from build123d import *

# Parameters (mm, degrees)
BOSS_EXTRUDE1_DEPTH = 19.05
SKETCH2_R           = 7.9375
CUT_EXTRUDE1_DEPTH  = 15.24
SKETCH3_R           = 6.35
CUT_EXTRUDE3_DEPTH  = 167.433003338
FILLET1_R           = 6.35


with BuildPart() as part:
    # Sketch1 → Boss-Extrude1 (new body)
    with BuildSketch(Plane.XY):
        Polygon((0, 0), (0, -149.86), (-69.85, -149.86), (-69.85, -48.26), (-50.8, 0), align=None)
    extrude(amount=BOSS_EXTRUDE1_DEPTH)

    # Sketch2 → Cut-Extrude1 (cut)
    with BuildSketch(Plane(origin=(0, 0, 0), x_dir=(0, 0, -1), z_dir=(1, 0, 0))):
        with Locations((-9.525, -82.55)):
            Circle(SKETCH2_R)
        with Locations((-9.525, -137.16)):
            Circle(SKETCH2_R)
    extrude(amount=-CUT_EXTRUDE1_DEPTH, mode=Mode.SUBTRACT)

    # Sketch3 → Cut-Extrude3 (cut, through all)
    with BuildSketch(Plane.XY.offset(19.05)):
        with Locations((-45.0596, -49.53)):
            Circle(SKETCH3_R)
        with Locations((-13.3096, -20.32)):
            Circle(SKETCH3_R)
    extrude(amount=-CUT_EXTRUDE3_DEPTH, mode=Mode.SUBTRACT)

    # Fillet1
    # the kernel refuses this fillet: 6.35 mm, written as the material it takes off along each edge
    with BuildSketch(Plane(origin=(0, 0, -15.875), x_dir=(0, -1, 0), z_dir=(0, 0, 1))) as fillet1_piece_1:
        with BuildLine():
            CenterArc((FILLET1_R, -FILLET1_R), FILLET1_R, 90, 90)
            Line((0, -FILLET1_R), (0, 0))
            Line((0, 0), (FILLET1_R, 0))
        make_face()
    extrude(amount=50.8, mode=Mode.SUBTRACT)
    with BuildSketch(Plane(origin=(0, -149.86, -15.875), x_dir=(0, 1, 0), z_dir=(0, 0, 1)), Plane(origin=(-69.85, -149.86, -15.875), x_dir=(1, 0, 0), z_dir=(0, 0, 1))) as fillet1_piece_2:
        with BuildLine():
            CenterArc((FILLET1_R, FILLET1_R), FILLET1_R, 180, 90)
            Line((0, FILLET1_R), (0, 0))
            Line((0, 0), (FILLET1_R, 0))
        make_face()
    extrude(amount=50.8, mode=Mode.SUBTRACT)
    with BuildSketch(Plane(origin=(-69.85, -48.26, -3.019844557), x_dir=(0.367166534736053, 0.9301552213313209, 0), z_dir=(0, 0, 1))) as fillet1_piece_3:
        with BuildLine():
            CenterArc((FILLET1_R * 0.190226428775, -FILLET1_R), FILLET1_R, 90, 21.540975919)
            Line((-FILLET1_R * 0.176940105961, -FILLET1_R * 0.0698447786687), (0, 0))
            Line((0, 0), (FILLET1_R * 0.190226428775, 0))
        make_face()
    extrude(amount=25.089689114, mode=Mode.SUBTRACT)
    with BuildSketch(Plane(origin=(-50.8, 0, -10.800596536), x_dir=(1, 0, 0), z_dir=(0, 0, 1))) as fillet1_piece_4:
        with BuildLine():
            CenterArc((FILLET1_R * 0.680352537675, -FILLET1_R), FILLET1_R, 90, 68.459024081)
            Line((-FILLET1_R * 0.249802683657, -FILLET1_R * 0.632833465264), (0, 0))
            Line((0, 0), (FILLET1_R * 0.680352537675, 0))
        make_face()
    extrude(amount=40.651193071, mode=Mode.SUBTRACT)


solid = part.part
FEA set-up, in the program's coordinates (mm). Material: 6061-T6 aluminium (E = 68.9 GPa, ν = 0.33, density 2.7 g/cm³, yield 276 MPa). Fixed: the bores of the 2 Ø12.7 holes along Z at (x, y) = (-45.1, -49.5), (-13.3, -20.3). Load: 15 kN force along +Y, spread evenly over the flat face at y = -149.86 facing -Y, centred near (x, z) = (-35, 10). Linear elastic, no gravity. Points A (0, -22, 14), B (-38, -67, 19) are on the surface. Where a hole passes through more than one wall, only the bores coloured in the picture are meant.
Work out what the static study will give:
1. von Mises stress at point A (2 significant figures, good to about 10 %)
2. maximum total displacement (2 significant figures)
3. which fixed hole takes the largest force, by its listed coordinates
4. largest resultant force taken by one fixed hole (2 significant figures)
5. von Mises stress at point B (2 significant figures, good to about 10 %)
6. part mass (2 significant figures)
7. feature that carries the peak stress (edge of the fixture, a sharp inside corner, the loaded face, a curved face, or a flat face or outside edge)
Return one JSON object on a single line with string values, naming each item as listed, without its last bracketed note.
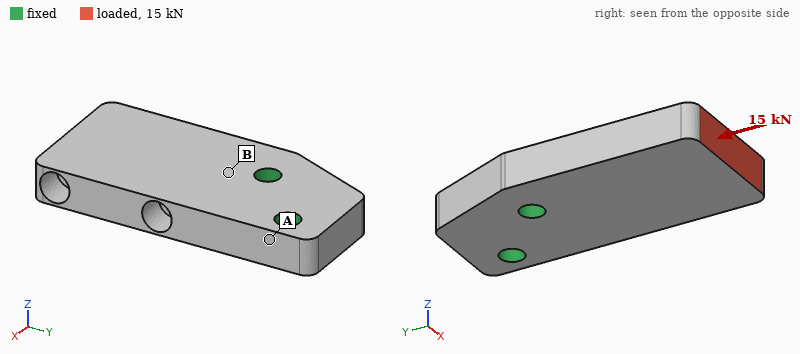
{"von Mises stress at point A": "6.1 MPa", "maximum total displacement": "36 µm", "which fixed hole takes the largest force, by its listed coordinates": "(-45.1, -49.5)", "largest resultant force taken by one fixed hole": "10 kN", "von Mises stress at point B": "17 MPa", "part mass": "480 g", "feature that carries the peak stress": "a curved face"}
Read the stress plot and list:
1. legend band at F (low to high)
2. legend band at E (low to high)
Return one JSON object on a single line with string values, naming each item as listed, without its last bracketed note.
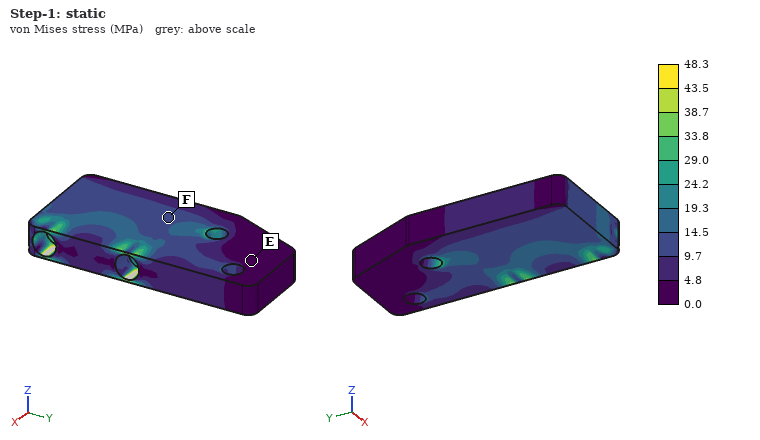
{"legend band at F": "9.7 to 14.5 MPa", "legend band at E": "0.0 to 4.8 MPa"}
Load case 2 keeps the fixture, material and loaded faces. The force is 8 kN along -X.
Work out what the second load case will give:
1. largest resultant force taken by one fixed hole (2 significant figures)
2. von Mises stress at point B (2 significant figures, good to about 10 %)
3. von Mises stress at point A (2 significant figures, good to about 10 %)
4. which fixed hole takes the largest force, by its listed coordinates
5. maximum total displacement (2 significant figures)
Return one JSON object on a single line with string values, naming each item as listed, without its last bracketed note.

{"largest resultant force taken by one fixed hole": "19 kN", "von Mises stress at point B": "19 MPa", "von Mises stress at point A": "18 MPa", "which fixed hole takes the largest force, by its listed coordinates": "(-45.1, -49.5)", "maximum total displacement": "0.19 mm"}
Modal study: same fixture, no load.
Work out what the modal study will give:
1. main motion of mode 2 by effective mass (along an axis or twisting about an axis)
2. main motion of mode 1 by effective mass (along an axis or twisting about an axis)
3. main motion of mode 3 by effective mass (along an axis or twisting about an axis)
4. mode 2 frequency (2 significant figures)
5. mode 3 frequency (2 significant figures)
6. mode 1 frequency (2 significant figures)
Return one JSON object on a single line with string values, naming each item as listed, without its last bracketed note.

{"main motion of mode 2 by effective mass": "along X", "main motion of mode 1 by effective mass": "along Z", "main motion of mode 3 by effective mass": "twisting about Y", "mode 2 frequency": "3300 Hz", "mode 3 frequency": "3800 Hz", "mode 1 frequency": "1500 Hz"}
